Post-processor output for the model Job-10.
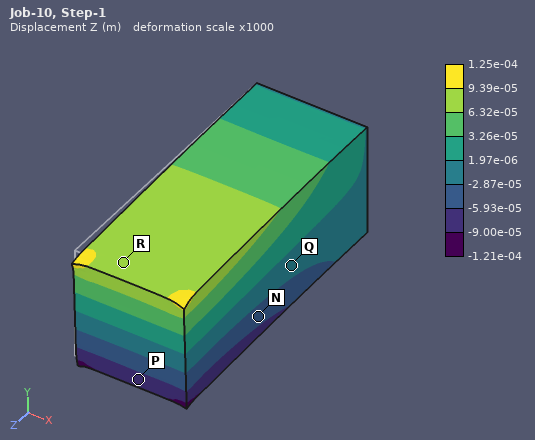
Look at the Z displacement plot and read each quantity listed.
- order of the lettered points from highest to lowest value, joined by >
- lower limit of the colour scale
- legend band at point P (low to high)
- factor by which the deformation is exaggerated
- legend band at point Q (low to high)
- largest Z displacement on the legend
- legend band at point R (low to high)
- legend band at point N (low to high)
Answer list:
R > Q > N > P
-1.21e-04 m
-9.00e-05 to -5.93e-05 m
1000
-2.87e-05 to 1.97e-06 m
1.25e-04 m
6.32e-05 to 9.39e-05 m
-5.93e-05 to -2.87e-05 m
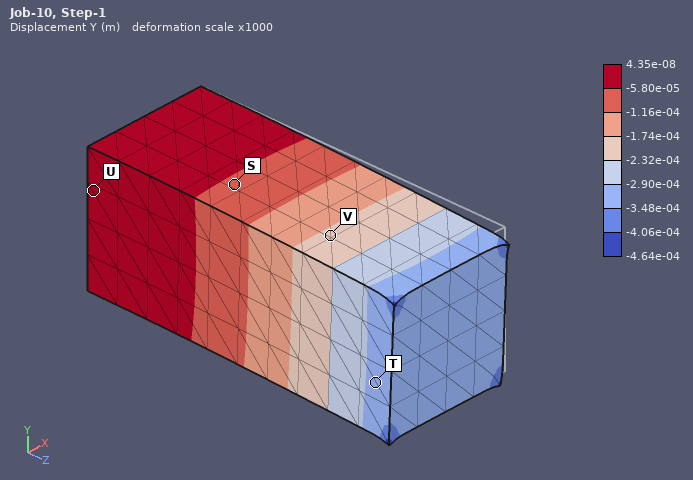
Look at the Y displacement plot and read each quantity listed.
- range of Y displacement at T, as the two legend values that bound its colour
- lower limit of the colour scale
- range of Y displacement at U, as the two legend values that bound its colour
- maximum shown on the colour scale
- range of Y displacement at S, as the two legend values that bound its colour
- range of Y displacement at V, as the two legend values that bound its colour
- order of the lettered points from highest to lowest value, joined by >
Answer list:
-3.48e-04 to -2.90e-04 m
-4.64e-04 m
-5.80e-05 to 4.35e-08 m
4.35e-08 m
-1.16e-04 to -5.80e-05 m
-2.32e-04 to -1.74e-04 m
U > S > V > T
